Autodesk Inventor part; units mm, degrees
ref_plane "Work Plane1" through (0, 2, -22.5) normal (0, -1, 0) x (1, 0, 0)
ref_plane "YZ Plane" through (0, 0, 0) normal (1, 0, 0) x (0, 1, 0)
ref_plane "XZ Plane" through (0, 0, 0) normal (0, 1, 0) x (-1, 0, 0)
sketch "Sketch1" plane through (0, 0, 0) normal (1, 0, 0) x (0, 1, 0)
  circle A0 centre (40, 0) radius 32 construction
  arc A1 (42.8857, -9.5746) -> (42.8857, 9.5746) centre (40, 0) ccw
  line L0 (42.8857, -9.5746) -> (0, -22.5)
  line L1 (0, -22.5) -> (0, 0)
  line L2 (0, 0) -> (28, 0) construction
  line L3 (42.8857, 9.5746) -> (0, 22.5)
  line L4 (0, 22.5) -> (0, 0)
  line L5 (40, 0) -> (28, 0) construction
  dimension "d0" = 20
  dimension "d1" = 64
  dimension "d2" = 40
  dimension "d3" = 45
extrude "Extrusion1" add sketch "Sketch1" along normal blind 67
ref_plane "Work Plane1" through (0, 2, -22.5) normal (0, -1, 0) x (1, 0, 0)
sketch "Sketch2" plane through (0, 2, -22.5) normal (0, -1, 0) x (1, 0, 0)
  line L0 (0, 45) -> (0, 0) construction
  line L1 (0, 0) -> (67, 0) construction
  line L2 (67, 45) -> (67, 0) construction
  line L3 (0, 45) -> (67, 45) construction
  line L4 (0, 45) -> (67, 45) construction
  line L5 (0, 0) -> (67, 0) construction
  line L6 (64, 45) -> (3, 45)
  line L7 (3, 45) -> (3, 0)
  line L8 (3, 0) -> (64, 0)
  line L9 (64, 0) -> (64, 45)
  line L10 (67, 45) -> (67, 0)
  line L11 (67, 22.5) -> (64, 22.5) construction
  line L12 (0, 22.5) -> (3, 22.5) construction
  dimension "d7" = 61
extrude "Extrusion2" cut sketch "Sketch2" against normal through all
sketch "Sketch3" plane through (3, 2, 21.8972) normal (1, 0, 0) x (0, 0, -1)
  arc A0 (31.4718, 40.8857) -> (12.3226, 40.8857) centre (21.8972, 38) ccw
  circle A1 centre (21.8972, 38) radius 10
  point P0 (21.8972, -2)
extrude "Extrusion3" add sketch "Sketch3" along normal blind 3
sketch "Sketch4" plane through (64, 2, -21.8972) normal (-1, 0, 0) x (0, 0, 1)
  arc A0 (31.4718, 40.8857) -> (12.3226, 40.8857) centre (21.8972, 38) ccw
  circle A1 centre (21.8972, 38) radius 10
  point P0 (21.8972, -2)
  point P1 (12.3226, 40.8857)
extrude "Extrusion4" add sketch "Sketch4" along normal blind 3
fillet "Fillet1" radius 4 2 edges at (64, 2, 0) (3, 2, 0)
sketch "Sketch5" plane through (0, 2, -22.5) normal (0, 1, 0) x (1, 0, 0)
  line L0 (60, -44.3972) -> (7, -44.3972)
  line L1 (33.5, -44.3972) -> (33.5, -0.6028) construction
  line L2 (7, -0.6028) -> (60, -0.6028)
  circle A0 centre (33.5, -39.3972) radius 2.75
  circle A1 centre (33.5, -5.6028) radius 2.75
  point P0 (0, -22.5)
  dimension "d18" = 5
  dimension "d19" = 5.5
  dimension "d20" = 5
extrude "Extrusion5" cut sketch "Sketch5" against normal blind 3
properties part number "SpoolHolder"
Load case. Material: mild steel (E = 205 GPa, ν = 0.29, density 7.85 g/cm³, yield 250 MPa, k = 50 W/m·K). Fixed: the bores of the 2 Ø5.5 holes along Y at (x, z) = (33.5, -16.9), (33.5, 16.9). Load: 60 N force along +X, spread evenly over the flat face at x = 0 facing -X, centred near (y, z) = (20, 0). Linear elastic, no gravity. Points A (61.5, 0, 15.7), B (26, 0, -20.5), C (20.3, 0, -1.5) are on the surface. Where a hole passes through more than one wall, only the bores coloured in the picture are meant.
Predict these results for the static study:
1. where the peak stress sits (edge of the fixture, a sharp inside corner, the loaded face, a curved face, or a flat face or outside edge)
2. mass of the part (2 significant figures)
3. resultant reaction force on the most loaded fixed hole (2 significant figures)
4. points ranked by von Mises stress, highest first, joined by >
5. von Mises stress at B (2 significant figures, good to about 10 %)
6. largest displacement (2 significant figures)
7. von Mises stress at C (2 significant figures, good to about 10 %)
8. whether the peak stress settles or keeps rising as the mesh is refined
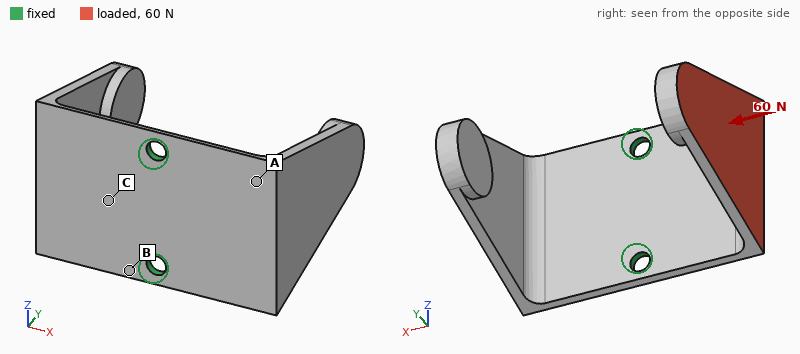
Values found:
edge of the fixture
130 g
31 N
B > C > A
45 MPa
0.30 mm
33 MPa
keeps rising
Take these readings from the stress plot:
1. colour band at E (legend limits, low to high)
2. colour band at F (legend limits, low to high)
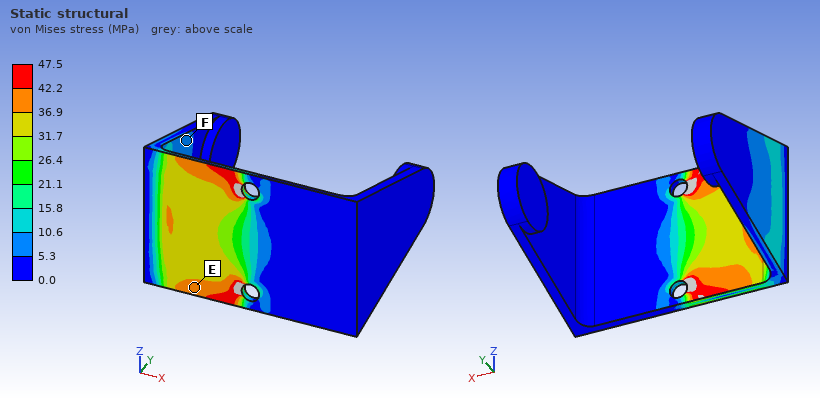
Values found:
36.9 to 42.2 MPa
5.3 to 10.6 MPa
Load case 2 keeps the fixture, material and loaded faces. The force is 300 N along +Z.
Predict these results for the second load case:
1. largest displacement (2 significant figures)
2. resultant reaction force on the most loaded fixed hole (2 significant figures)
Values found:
0.35 mm
360 N
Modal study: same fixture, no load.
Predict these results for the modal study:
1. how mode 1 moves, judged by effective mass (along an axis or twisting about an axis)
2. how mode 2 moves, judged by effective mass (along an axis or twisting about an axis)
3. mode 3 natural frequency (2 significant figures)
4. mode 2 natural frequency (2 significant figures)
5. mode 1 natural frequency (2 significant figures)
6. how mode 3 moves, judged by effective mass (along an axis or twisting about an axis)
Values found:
along X
along Y
760 Hz
350 Hz
340 Hz
twisting about Y
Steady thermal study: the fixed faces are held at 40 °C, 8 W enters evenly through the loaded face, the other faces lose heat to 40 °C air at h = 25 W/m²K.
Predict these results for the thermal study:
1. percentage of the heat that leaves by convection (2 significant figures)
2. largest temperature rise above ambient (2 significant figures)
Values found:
47 %
52 K
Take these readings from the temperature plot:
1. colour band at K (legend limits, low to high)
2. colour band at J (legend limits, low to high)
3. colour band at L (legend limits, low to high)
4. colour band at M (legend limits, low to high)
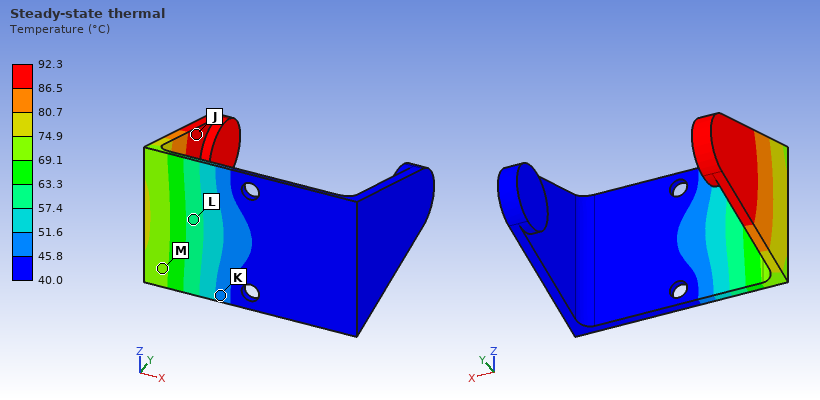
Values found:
45.8 to 51.6 °C
86.5 to 92.3 °C
57.4 to 63.3 °C
69.1 to 74.9 °C
